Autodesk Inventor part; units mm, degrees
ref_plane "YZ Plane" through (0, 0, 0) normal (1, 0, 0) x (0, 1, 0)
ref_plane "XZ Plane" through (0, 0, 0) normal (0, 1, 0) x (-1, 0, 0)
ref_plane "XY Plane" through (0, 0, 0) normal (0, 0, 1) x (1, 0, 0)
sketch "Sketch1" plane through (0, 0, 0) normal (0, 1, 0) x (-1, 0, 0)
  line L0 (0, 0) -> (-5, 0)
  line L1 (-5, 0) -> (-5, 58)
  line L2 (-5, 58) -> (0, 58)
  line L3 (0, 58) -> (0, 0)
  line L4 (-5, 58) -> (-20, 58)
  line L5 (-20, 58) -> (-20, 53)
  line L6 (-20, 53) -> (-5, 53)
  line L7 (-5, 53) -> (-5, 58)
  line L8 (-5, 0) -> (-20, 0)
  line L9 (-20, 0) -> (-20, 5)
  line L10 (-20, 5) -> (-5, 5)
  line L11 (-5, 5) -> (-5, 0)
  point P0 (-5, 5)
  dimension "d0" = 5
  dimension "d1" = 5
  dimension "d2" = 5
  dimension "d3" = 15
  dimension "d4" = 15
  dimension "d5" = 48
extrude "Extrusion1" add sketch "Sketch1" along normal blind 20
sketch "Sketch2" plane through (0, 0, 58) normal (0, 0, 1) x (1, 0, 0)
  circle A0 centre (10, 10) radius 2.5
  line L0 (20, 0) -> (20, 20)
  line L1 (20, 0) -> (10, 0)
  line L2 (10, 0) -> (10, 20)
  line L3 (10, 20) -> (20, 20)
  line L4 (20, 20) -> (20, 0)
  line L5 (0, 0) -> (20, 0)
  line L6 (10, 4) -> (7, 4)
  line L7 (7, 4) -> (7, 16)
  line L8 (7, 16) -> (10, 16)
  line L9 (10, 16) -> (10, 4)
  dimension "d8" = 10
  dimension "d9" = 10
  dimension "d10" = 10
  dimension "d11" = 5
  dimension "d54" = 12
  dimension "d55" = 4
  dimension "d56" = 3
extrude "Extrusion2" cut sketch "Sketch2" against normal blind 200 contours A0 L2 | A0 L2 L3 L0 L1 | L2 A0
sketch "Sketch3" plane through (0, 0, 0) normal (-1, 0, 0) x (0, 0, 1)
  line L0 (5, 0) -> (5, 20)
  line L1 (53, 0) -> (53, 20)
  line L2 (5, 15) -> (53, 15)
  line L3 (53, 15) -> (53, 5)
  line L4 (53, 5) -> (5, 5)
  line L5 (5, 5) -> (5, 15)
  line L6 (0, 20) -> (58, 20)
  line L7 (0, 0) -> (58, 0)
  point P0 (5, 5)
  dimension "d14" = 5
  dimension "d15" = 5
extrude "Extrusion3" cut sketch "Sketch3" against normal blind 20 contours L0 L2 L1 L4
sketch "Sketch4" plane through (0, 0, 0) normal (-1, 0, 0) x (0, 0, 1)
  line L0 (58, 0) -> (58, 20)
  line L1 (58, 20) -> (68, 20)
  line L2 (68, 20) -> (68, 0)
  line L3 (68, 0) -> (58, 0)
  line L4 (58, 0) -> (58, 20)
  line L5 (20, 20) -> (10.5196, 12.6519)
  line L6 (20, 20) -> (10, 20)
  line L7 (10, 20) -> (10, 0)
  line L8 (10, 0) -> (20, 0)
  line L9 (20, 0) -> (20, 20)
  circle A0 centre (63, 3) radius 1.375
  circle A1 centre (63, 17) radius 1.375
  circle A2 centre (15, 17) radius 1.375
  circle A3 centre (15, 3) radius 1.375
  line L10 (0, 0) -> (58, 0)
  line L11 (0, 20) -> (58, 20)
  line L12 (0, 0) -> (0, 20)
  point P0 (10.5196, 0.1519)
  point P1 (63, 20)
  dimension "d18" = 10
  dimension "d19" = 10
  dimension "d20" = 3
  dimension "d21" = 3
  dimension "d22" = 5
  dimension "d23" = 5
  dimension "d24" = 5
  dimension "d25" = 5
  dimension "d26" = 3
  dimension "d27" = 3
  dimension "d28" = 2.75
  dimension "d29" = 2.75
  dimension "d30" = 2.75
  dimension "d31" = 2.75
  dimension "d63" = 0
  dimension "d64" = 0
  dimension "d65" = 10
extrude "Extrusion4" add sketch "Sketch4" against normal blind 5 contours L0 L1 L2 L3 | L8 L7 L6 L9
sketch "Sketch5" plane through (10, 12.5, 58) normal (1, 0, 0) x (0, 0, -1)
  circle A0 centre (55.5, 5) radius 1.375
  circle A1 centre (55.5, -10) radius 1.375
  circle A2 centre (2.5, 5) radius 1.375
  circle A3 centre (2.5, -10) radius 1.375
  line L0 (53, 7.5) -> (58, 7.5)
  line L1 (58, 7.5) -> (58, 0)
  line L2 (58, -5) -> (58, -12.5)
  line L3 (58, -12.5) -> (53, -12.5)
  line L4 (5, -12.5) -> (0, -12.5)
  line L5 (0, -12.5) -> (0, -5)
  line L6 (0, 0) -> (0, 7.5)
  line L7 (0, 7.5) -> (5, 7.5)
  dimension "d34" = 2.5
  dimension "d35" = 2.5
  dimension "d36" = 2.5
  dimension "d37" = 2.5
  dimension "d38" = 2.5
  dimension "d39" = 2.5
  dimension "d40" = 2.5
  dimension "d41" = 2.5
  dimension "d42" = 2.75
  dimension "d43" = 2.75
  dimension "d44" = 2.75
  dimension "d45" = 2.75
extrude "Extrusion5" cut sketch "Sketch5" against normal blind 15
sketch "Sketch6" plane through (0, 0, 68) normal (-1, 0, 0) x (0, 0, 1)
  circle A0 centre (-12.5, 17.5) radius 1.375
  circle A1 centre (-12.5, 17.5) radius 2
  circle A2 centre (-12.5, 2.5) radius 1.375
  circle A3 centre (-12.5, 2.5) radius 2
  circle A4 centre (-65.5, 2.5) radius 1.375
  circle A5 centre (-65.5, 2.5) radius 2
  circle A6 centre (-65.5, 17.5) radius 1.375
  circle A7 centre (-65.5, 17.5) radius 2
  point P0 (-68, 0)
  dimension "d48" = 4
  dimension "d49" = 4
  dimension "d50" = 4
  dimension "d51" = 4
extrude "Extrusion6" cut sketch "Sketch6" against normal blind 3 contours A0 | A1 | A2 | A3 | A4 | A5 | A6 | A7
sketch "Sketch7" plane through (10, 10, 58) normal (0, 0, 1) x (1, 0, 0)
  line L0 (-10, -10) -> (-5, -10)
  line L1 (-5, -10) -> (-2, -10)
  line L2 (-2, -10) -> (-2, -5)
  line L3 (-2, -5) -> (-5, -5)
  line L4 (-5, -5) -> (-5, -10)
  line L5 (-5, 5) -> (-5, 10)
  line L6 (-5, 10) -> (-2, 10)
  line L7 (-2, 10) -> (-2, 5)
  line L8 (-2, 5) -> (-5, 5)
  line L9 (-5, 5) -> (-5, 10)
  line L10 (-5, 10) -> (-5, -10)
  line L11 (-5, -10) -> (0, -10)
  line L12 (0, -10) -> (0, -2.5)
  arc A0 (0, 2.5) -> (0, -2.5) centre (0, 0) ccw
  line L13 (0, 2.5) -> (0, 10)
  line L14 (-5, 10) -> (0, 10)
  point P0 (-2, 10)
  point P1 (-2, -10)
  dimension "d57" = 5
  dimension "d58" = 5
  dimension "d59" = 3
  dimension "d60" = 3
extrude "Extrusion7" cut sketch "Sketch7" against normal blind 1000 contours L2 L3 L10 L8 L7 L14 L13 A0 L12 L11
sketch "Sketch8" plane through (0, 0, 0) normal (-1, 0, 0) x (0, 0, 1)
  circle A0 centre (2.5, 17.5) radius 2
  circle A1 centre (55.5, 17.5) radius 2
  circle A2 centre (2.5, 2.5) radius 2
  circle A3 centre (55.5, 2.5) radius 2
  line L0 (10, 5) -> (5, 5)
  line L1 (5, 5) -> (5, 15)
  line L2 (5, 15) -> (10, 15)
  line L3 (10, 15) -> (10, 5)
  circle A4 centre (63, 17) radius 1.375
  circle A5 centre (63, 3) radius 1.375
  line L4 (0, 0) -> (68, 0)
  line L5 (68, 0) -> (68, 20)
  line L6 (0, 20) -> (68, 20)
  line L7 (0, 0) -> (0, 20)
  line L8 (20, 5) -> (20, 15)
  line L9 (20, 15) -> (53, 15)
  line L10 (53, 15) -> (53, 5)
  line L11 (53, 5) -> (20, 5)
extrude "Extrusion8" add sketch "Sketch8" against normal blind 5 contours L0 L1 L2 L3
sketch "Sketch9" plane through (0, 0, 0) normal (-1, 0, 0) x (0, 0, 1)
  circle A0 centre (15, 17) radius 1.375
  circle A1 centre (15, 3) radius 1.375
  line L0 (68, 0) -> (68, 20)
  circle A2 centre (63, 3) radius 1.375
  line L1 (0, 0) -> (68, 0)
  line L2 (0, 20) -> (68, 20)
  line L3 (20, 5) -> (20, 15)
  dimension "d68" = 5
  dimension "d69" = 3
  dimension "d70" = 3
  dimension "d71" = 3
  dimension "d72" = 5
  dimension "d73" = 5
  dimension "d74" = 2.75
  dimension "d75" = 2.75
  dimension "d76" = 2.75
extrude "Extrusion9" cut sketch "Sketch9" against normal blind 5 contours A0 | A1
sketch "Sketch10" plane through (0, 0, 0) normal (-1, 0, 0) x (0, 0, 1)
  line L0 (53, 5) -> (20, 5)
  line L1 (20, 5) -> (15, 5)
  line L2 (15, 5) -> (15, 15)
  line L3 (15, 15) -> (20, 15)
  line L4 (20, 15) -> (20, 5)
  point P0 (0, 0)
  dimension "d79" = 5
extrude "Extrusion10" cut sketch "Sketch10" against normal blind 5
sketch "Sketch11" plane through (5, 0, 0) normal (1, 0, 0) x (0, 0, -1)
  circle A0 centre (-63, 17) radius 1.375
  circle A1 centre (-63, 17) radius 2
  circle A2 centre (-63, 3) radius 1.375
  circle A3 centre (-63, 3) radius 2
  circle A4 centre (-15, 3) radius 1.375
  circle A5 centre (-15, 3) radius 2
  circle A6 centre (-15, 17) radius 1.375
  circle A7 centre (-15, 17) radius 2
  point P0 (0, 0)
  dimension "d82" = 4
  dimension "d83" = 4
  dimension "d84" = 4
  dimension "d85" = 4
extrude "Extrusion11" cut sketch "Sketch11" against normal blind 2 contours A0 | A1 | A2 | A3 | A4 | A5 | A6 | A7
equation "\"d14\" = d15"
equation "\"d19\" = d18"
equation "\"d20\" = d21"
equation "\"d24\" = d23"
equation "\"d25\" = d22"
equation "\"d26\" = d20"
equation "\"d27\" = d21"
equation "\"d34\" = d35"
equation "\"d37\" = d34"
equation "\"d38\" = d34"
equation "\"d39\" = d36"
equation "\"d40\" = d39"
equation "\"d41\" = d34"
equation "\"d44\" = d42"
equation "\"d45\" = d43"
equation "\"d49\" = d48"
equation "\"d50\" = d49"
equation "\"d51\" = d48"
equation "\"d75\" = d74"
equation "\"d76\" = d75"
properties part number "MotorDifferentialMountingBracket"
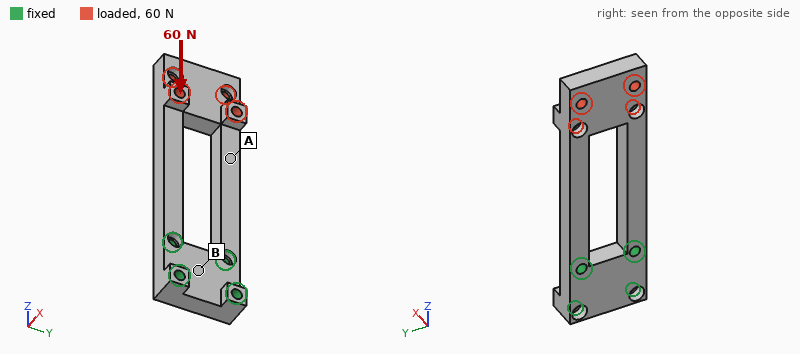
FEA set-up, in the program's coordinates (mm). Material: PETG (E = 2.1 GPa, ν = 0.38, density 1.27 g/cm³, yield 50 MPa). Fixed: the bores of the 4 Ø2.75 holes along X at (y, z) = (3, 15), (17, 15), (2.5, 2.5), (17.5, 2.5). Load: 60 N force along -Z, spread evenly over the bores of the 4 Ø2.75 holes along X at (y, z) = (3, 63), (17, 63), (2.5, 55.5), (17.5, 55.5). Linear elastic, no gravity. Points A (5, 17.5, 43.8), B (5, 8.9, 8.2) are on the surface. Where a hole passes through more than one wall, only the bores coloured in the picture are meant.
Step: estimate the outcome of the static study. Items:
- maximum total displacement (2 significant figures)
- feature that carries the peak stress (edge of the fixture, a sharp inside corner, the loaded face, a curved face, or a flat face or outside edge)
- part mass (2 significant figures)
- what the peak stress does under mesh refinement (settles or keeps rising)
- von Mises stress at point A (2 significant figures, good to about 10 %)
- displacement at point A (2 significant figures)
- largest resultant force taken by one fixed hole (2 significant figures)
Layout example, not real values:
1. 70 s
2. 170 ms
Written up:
1. 0.67 mm
2. a sharp inside corner
3. 6.0 g
4. keeps rising
5. 3.4 MPa
6. 0.25 mm
7. 27 N
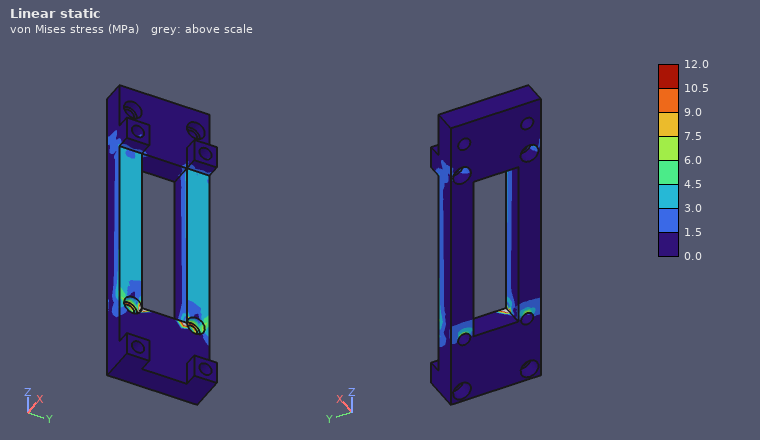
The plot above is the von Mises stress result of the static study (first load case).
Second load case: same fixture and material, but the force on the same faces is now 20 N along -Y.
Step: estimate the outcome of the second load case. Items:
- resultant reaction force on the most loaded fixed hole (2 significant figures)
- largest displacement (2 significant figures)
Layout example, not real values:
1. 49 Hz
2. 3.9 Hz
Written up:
1. 29 N
2. 0.73 mm
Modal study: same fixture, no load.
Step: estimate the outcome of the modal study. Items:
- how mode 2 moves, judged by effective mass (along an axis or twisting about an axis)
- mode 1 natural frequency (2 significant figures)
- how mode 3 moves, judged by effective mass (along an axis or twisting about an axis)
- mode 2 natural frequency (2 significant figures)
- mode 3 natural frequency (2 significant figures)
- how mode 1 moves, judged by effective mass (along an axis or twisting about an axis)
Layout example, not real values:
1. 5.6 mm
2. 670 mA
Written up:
1. along Y
2. 260 Hz
3. twisting about Z
4. 530 Hz
5. 1000 Hz
6. along X
